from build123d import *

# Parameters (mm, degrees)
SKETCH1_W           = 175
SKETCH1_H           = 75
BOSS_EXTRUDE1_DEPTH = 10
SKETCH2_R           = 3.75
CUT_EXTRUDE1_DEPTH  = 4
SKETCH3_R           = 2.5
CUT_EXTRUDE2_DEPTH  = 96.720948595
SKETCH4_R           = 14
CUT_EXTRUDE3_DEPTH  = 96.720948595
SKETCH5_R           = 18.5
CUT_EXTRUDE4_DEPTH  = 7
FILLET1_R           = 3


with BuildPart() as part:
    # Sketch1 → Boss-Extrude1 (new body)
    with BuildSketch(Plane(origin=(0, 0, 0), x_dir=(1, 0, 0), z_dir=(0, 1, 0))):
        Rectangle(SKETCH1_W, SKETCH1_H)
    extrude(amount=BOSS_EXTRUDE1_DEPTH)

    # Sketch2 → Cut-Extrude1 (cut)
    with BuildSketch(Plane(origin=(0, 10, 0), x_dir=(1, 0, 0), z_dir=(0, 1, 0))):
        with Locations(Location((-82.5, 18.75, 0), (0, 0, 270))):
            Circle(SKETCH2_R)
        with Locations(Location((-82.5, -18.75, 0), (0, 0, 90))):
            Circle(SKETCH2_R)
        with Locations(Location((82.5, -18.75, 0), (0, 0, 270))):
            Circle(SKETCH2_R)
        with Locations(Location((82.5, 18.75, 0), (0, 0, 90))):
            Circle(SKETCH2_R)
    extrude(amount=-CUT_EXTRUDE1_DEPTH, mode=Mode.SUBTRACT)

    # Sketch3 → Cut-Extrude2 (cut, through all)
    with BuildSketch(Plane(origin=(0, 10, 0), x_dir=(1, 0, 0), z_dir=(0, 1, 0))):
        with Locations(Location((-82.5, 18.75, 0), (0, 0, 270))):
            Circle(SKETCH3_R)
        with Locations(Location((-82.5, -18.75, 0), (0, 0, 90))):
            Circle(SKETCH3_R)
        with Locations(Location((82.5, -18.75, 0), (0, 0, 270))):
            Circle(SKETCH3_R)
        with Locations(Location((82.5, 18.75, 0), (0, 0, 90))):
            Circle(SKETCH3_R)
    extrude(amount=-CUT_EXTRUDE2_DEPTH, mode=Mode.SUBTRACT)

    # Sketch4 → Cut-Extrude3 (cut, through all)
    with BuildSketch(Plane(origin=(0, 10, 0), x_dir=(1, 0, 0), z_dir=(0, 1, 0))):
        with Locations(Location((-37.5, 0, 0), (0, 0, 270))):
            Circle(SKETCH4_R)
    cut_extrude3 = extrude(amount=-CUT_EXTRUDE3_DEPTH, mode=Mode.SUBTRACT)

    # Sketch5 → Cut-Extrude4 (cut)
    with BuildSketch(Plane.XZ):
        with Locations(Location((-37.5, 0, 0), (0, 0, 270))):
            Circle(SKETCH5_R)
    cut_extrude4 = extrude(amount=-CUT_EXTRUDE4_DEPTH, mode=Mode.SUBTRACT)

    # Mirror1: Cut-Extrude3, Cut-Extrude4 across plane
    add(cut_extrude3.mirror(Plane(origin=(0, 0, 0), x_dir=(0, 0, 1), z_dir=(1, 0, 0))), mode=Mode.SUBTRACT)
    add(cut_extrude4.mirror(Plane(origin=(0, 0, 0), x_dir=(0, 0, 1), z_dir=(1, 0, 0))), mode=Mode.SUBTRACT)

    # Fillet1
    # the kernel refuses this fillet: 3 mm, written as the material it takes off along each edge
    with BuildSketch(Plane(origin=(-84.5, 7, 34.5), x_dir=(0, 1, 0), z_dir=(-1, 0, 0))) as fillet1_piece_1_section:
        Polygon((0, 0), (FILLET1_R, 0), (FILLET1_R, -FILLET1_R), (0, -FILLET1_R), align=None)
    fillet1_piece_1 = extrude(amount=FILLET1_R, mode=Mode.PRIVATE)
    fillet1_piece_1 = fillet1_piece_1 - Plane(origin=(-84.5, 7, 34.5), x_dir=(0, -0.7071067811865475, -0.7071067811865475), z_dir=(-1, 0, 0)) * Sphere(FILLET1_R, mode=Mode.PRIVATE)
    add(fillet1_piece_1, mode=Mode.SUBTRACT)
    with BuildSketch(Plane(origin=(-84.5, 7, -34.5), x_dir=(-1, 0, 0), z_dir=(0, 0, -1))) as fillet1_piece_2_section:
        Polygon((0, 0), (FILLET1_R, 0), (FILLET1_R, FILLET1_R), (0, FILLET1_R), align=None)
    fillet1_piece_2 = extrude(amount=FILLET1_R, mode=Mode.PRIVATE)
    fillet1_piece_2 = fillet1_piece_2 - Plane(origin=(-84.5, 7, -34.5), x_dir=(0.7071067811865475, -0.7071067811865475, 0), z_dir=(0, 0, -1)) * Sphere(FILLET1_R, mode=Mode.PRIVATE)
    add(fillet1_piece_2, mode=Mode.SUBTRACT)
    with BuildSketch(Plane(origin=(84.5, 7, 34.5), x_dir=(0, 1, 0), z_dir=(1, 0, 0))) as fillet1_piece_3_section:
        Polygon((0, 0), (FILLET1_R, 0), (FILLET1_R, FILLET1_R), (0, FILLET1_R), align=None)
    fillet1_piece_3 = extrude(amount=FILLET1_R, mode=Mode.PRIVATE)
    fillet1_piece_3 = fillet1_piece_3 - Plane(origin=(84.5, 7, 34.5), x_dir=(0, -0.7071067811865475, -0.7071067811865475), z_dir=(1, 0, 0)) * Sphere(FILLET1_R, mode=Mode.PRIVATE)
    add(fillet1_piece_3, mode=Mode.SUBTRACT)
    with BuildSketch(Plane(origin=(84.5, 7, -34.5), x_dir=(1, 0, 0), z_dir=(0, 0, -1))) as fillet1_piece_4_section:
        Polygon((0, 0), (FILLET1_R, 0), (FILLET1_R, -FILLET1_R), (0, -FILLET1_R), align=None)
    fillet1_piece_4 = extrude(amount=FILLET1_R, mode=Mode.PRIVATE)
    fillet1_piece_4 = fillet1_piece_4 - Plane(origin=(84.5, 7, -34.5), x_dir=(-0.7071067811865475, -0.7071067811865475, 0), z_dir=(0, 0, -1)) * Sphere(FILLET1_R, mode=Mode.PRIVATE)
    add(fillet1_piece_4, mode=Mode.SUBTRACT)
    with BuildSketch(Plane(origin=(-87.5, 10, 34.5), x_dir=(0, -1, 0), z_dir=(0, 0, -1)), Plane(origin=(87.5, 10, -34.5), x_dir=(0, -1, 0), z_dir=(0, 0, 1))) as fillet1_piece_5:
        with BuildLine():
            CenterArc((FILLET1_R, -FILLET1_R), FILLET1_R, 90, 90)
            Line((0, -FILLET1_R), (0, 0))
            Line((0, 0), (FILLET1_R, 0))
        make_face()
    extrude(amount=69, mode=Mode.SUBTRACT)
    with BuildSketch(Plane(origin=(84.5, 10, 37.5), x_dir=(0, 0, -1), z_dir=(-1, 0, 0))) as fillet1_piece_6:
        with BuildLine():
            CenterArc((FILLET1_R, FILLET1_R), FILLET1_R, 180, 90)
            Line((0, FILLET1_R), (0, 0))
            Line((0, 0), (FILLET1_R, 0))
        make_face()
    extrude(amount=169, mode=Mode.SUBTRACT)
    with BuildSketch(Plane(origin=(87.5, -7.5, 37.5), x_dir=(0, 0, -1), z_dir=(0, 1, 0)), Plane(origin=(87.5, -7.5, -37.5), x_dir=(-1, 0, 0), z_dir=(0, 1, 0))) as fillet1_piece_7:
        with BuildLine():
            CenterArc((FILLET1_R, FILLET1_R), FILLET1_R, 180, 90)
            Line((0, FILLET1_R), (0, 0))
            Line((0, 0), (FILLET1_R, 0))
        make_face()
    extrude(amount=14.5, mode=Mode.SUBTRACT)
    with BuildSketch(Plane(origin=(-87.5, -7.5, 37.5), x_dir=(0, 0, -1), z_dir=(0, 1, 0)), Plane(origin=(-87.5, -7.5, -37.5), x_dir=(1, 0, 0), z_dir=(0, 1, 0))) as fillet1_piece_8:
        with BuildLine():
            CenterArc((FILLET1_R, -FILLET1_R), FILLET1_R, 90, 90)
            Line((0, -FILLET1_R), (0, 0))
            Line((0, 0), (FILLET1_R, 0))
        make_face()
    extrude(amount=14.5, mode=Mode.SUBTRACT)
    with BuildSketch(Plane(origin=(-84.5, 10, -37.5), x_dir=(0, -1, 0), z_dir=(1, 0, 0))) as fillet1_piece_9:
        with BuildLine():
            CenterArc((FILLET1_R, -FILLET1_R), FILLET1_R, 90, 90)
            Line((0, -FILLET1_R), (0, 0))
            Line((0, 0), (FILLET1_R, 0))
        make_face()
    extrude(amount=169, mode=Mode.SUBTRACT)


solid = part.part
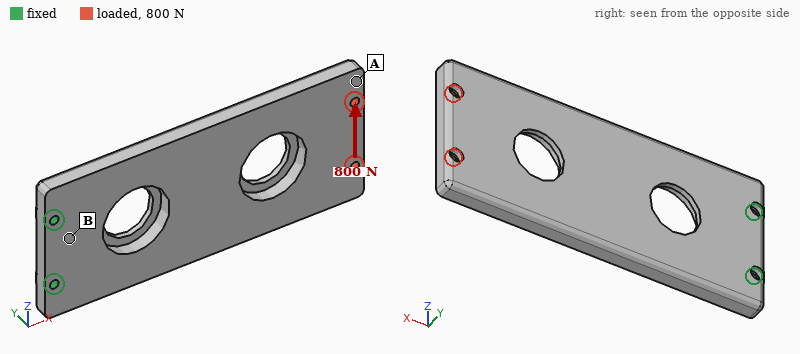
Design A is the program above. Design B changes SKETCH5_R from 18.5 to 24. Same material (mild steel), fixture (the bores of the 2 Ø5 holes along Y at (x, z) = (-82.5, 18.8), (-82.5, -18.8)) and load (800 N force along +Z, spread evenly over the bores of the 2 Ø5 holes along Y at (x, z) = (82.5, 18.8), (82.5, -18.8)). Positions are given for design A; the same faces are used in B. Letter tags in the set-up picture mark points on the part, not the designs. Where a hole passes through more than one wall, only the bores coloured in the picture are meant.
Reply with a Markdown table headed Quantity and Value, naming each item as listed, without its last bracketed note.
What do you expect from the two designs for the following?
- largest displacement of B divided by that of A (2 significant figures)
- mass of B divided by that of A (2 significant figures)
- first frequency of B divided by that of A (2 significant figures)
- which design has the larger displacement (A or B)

| Quantity | Value |
|---|---|
| largest displacement of B divided by that of A | 1.2 |
| mass of B divided by that of A | 0.91 |
| first frequency of B divided by that of A | 0.98 |
| which design has the larger displacement | B |
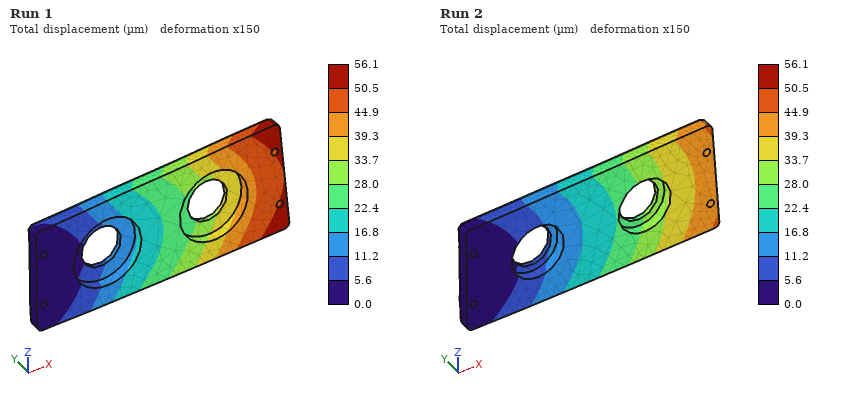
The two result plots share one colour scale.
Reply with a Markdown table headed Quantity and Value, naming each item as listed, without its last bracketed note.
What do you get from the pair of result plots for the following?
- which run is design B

| Quantity | Value |
|---|---|
| which run is design B | Run 1 |
